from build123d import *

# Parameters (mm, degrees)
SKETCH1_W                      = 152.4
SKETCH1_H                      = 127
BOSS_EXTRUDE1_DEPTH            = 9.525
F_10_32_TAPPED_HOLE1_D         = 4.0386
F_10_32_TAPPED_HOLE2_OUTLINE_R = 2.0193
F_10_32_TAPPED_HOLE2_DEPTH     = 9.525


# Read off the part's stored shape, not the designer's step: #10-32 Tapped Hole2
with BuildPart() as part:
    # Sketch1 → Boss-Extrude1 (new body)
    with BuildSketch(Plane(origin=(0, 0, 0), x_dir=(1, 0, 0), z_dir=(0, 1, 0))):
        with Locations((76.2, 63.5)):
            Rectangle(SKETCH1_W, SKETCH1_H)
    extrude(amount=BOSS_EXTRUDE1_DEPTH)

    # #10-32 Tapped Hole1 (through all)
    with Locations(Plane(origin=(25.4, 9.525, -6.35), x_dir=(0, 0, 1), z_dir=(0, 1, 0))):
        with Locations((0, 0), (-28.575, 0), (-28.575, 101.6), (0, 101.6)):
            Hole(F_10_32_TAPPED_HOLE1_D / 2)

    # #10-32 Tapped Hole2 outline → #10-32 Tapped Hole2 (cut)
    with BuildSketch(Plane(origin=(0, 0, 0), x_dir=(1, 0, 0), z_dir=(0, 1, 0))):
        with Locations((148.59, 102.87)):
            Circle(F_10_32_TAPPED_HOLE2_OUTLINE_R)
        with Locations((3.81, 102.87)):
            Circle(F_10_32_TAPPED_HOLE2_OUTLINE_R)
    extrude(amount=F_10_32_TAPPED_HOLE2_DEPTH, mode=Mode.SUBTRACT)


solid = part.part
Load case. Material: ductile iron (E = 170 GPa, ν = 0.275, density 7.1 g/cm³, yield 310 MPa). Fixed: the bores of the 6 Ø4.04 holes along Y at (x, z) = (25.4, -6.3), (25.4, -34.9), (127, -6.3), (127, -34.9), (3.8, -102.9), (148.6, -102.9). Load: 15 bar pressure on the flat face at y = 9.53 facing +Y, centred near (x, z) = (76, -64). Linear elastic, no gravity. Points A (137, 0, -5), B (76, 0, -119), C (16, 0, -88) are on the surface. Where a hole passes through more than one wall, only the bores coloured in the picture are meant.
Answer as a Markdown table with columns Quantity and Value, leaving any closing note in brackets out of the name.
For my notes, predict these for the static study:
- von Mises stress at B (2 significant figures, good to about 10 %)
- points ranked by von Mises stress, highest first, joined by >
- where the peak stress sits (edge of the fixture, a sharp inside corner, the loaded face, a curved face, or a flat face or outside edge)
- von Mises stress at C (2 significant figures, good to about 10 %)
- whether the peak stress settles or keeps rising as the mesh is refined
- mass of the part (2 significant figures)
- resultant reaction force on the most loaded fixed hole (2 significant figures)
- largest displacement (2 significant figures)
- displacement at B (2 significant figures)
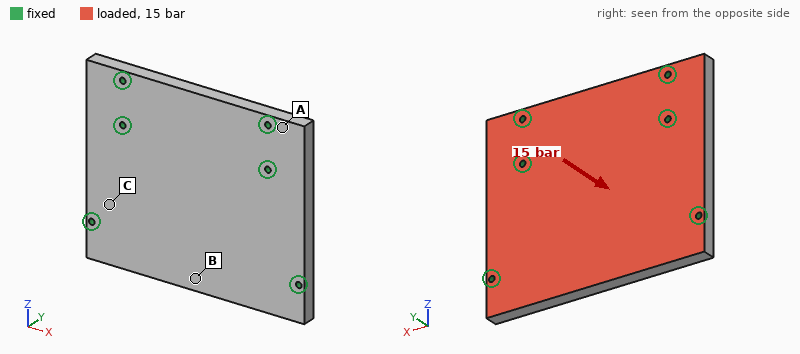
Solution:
| Quantity | Value |
|---|---|
| von Mises stress at B | 97 MPa |
| points ranked by von Mises stress, highest first, joined by > | B > C > A |
| where the peak stress sits | edge of the fixture |
| von Mises stress at C | 53 MPa |
| whether the peak stress settles or keeps rising as the mesh is refined | keeps rising |
| mass of the part | 1.3 kg |
| resultant reaction force on the most loaded fixed hole | 7.3 kN |
| largest displacement | 0.23 mm |
| displacement at B | 0.22 mm |
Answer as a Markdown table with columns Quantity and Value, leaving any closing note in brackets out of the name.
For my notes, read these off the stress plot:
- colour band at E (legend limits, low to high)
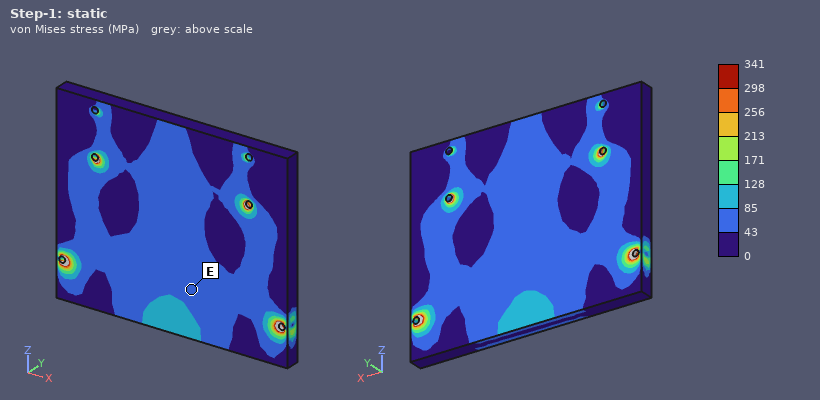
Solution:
| Quantity | Value |
|---|---|
| colour band at E | 43 to 85 MPa |
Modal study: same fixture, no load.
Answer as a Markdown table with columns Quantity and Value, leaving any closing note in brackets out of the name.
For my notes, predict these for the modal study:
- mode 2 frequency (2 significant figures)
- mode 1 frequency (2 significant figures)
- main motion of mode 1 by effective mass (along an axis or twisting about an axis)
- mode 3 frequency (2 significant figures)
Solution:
| Quantity | Value |
|---|---|
| mode 2 frequency | 4000 Hz |
| mode 1 frequency | 2000 Hz |
| main motion of mode 1 by effective mass | along Y |
| mode 3 frequency | 5200 Hz |
